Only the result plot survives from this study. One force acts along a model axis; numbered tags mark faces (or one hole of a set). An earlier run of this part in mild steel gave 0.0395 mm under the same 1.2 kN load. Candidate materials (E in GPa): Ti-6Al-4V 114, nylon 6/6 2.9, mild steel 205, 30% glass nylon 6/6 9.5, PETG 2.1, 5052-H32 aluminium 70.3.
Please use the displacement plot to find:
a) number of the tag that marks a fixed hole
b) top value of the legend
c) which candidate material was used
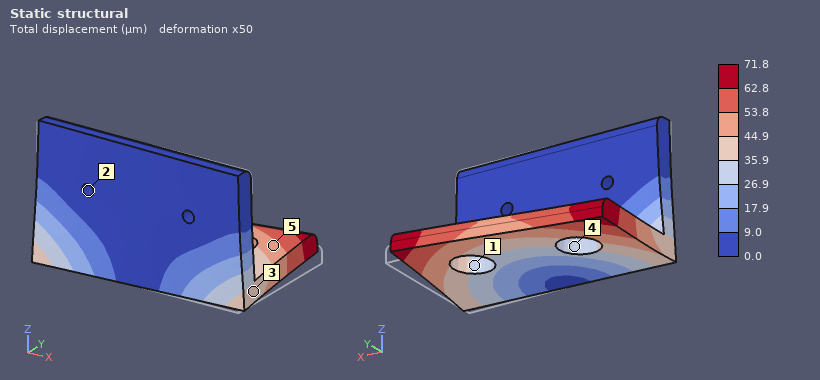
2
71.8 µm
Ti-6Al-4V
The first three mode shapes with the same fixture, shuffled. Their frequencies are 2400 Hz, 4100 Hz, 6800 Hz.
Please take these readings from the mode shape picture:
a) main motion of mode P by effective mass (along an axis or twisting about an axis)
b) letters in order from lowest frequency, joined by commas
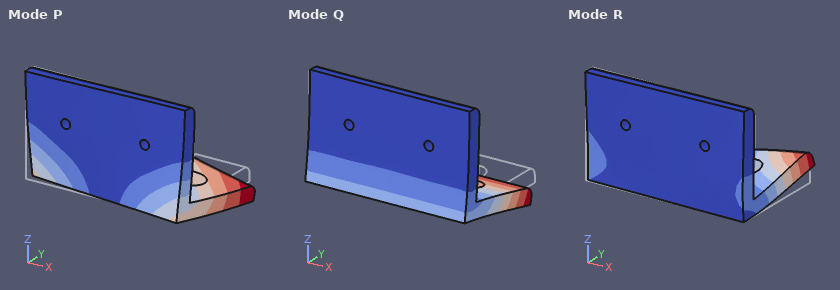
along X
Q, P, R
